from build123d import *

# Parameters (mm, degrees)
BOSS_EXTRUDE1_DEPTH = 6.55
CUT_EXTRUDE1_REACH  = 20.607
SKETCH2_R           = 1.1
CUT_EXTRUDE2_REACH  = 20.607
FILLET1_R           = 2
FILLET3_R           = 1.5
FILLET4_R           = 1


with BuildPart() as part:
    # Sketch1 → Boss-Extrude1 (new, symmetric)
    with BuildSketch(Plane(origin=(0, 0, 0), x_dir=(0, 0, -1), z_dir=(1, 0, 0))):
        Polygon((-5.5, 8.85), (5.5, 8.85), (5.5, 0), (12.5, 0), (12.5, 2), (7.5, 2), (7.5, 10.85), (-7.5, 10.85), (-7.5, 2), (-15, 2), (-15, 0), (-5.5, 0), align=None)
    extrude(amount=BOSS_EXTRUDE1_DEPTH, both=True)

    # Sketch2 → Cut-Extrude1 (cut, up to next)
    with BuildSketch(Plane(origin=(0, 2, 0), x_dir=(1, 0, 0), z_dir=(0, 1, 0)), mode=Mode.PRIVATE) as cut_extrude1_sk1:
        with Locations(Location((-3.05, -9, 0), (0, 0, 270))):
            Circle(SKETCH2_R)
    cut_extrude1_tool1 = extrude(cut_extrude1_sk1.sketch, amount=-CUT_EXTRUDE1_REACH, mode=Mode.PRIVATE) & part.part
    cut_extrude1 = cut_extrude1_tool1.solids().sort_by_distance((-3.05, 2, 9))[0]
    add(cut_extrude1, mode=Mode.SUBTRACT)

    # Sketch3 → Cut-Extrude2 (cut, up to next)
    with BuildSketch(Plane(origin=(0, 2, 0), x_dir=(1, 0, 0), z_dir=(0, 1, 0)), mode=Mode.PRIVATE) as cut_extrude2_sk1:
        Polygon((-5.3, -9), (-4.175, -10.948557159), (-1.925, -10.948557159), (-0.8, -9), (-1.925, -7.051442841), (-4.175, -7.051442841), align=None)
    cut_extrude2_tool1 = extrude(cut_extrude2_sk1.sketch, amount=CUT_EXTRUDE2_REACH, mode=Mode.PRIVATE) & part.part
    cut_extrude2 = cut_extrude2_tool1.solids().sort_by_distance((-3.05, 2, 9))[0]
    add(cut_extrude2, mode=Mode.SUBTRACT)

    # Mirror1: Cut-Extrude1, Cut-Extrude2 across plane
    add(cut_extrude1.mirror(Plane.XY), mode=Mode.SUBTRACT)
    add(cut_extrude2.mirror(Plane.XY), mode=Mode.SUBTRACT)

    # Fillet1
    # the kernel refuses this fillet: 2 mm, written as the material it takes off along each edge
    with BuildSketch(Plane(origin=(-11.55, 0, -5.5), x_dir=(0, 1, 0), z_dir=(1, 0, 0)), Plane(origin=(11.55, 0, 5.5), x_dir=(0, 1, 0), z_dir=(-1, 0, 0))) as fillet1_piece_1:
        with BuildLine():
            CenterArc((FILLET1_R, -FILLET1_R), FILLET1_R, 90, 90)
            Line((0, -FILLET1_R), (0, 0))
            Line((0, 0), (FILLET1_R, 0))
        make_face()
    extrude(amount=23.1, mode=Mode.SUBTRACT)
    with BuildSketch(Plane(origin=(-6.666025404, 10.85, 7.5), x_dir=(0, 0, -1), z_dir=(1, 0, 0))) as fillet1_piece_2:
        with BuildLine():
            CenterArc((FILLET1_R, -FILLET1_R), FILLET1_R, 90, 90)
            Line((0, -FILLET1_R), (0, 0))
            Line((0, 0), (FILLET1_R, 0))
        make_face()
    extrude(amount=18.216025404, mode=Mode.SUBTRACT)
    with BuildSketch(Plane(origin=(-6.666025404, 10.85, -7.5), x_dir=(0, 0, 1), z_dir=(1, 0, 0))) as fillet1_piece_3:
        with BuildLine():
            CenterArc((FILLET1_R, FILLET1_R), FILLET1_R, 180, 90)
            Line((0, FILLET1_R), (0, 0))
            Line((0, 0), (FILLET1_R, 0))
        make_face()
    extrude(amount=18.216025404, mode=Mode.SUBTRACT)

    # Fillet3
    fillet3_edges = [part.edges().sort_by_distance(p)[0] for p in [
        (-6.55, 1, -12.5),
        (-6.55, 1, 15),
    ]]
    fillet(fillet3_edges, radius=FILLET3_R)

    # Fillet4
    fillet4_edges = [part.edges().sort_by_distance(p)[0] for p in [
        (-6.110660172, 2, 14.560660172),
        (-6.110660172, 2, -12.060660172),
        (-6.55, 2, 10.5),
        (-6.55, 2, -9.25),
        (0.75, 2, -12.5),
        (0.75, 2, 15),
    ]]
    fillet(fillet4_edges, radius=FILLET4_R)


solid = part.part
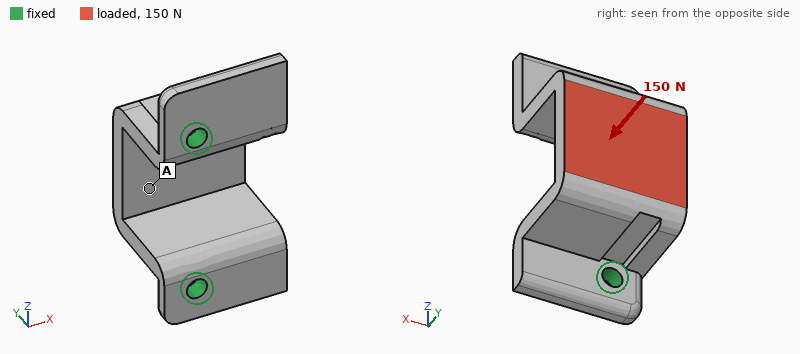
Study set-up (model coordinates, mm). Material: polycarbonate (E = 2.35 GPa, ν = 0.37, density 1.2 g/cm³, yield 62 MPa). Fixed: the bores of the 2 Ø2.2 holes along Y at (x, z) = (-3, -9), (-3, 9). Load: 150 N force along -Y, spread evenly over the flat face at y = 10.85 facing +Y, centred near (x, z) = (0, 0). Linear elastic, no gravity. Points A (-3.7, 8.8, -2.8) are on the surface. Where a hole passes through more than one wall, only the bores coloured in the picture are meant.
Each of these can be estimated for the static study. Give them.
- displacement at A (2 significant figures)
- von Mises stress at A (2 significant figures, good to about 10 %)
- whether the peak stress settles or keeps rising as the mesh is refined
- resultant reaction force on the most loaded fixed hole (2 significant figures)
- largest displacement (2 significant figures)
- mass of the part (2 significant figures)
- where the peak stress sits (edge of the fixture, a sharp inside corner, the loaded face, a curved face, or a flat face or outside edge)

0.18 mm
7.5 MPa
keeps rising
80 N
0.39 mm
1.3 g
edge of the fixture
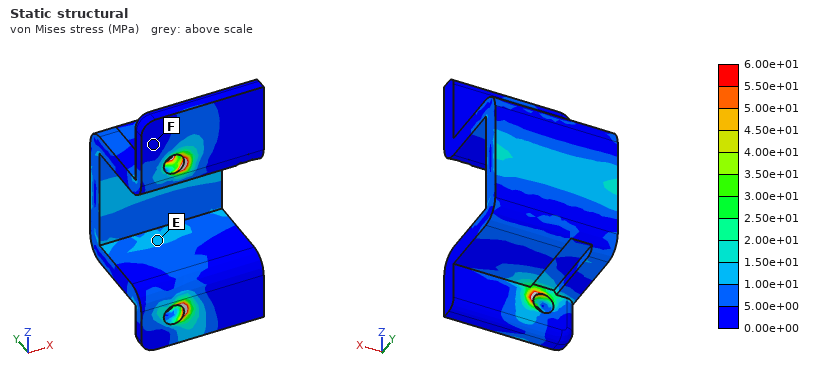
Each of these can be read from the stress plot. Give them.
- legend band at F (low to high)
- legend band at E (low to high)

0.00e+00 to 5.00e+00 MPa
1.00e+01 to 1.50e+01 MPa
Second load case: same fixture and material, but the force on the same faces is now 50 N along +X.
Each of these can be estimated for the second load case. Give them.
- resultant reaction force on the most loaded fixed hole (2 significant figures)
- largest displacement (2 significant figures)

25 N
0.35 mm
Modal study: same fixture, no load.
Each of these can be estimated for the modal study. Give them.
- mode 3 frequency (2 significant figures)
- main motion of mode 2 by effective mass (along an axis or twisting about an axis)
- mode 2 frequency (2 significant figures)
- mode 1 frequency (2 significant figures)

4600 Hz
along Z
3600 Hz
2700 Hz
